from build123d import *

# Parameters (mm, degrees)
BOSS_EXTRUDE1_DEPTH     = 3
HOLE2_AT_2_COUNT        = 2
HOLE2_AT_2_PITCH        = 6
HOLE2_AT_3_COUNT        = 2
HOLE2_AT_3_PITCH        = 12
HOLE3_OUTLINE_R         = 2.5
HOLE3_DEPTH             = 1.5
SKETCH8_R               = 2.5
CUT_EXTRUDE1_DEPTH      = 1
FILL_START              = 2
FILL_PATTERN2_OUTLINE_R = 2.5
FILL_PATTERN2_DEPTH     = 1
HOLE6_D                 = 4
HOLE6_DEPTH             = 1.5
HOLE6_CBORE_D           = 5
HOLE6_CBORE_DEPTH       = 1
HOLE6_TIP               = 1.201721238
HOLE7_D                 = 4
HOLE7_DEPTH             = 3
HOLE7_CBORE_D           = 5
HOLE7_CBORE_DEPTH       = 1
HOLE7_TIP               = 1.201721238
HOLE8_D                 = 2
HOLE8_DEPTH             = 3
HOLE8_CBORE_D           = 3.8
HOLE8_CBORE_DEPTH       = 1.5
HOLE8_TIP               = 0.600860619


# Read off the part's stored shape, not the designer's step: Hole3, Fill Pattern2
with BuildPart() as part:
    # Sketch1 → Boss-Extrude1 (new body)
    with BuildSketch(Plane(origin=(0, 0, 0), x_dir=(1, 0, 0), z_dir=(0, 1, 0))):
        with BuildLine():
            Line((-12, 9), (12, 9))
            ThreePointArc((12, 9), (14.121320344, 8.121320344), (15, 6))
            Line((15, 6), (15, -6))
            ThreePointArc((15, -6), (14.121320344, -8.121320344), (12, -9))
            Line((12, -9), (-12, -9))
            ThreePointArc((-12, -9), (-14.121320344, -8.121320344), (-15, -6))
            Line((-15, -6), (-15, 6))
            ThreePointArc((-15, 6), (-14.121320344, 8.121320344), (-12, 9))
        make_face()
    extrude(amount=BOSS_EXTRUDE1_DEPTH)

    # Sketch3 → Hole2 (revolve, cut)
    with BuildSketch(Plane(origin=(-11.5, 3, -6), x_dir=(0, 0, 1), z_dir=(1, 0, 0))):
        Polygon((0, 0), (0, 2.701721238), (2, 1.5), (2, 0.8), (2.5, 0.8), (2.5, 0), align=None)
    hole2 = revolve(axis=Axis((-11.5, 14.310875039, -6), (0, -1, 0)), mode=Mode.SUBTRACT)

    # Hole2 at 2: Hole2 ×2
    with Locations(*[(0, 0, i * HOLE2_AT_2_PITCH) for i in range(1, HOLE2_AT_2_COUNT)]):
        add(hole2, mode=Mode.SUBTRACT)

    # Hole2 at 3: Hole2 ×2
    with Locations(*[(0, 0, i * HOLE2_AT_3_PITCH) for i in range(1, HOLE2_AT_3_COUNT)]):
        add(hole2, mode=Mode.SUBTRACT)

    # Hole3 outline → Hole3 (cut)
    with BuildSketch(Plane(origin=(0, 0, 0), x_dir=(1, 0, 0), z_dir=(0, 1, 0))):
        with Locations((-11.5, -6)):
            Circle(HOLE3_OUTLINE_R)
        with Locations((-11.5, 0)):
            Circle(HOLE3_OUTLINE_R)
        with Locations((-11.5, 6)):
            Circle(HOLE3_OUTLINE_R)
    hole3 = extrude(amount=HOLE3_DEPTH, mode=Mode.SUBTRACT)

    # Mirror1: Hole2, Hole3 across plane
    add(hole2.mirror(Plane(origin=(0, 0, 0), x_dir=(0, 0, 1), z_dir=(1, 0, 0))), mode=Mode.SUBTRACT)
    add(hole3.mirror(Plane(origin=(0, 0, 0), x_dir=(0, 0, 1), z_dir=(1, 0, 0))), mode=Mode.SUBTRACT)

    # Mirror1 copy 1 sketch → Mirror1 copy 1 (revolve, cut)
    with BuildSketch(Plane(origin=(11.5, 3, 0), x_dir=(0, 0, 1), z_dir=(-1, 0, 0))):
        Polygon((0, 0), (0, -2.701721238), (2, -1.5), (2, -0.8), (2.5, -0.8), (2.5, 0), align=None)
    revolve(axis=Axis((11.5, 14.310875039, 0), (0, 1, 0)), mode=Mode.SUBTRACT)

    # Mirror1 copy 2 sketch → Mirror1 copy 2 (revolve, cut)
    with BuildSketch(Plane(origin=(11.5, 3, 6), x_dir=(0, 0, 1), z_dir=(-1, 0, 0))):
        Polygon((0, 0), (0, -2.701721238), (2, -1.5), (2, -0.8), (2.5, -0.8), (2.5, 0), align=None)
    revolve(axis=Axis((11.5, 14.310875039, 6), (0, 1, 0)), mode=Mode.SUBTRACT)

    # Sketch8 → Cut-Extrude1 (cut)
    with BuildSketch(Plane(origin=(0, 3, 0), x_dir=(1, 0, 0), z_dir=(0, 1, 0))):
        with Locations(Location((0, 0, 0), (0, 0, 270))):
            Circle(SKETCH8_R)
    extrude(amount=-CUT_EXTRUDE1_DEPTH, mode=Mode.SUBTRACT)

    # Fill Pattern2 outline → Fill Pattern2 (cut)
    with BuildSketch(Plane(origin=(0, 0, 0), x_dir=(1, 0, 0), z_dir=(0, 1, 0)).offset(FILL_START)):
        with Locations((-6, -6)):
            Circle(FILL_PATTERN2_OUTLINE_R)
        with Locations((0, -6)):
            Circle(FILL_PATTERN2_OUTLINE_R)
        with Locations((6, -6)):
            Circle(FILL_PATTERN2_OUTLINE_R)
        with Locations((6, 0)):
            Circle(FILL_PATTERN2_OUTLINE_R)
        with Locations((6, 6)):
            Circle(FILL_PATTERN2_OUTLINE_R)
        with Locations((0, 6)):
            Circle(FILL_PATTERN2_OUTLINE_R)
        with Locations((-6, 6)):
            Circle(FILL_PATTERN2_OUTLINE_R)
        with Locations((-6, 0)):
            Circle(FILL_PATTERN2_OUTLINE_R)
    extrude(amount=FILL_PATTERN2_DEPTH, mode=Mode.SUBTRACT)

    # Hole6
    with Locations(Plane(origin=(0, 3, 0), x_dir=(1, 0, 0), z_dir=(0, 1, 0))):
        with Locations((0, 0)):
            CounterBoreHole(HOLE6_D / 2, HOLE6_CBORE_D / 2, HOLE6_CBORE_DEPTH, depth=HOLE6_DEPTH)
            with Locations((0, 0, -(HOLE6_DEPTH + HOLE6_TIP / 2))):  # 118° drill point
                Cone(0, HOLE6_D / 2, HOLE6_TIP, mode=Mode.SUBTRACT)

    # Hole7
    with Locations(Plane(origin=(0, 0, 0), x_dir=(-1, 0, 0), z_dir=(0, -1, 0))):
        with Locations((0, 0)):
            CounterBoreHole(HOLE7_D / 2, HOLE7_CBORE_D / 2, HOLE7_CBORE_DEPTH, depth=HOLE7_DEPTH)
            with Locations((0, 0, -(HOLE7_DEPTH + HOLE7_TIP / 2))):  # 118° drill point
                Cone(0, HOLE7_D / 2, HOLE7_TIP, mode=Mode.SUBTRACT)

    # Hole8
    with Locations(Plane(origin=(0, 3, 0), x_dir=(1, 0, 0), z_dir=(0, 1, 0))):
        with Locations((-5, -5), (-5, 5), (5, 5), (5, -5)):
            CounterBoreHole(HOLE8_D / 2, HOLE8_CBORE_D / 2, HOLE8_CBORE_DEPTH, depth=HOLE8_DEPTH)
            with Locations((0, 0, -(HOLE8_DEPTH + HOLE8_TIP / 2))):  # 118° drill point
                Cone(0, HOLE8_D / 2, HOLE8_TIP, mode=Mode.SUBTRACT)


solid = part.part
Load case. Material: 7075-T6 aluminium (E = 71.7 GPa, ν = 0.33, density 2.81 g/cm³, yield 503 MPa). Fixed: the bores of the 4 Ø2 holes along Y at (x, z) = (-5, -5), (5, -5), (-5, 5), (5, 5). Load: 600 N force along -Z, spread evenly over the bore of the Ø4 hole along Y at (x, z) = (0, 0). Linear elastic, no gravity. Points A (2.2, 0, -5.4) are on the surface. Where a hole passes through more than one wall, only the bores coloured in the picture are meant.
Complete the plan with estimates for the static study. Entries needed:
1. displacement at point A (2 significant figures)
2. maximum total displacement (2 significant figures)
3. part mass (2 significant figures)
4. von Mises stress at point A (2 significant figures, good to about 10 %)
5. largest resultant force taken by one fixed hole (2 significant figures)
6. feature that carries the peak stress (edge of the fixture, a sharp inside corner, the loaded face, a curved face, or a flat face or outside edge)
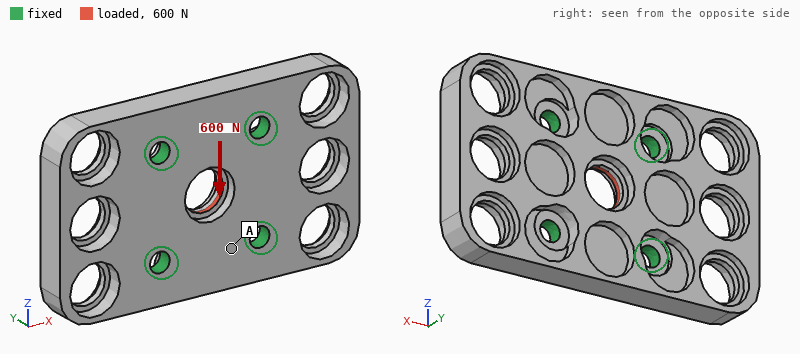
0.77 µm
2.7 µm
2.8 g
9.2 MPa
160 N
a sharp inside corner
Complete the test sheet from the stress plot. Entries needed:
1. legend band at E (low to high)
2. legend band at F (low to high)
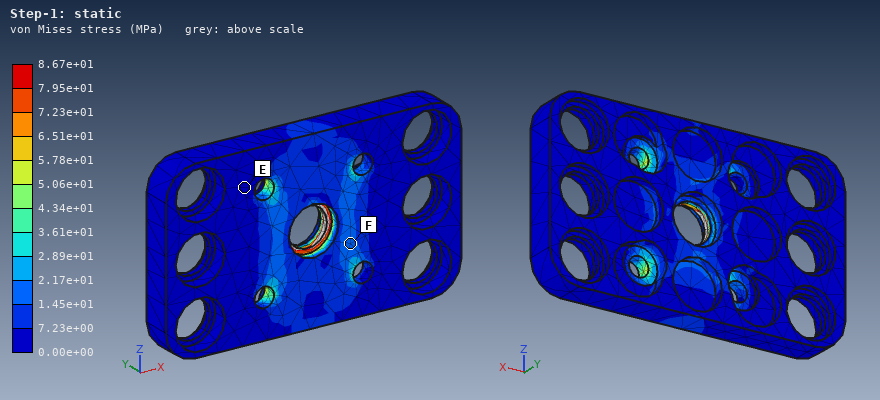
0.00e+00 to 7.23e+00 MPa
1.45e+01 to 2.17e+01 MPa
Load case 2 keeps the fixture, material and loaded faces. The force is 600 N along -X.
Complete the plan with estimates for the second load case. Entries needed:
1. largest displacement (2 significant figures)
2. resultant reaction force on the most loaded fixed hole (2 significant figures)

2.7 µm
160 N
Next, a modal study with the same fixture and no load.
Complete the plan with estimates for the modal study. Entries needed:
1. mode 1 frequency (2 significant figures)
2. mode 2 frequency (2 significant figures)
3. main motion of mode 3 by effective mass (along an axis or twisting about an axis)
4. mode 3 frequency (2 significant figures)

17 kHz
18 kHz
twisting about X
26 kHz
